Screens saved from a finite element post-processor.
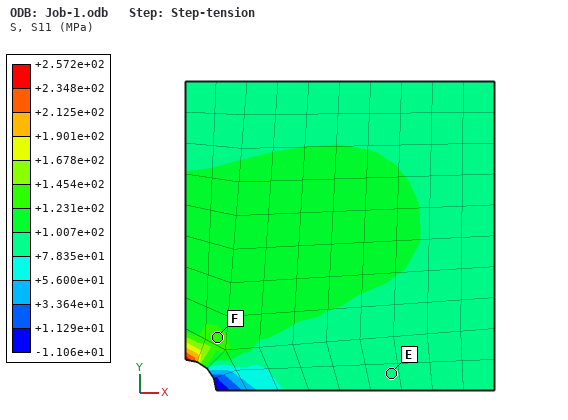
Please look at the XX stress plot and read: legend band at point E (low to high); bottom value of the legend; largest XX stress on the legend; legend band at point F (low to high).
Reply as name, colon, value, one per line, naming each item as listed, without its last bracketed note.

legend band at point E: +7.835e+01 to +1.007e+02 MPa
bottom value of the legend: -1.106e+01 MPa
largest XX stress on the legend: +2.572e+02 MPa
legend band at point F: +1.231e+02 to +1.454e+02 MPa
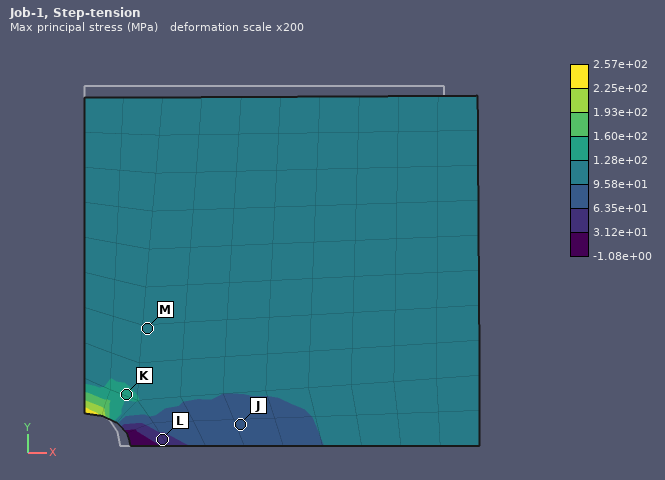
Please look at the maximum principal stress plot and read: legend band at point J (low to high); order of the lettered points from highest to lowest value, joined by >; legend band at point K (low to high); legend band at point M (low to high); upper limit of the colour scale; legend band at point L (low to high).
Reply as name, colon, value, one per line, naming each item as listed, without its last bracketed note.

legend band at point J: 6.35e+01 to 9.58e+01 MPa
order of the lettered points from highest to lowest value, joined by >: K > M > J > L
legend band at point K: 1.28e+02 to 1.60e+02 MPa
legend band at point M: 9.58e+01 to 1.28e+02 MPa
upper limit of the colour scale: 2.57e+02 MPa
legend band at point L: 3.12e+01 to 6.35e+01 MPa
